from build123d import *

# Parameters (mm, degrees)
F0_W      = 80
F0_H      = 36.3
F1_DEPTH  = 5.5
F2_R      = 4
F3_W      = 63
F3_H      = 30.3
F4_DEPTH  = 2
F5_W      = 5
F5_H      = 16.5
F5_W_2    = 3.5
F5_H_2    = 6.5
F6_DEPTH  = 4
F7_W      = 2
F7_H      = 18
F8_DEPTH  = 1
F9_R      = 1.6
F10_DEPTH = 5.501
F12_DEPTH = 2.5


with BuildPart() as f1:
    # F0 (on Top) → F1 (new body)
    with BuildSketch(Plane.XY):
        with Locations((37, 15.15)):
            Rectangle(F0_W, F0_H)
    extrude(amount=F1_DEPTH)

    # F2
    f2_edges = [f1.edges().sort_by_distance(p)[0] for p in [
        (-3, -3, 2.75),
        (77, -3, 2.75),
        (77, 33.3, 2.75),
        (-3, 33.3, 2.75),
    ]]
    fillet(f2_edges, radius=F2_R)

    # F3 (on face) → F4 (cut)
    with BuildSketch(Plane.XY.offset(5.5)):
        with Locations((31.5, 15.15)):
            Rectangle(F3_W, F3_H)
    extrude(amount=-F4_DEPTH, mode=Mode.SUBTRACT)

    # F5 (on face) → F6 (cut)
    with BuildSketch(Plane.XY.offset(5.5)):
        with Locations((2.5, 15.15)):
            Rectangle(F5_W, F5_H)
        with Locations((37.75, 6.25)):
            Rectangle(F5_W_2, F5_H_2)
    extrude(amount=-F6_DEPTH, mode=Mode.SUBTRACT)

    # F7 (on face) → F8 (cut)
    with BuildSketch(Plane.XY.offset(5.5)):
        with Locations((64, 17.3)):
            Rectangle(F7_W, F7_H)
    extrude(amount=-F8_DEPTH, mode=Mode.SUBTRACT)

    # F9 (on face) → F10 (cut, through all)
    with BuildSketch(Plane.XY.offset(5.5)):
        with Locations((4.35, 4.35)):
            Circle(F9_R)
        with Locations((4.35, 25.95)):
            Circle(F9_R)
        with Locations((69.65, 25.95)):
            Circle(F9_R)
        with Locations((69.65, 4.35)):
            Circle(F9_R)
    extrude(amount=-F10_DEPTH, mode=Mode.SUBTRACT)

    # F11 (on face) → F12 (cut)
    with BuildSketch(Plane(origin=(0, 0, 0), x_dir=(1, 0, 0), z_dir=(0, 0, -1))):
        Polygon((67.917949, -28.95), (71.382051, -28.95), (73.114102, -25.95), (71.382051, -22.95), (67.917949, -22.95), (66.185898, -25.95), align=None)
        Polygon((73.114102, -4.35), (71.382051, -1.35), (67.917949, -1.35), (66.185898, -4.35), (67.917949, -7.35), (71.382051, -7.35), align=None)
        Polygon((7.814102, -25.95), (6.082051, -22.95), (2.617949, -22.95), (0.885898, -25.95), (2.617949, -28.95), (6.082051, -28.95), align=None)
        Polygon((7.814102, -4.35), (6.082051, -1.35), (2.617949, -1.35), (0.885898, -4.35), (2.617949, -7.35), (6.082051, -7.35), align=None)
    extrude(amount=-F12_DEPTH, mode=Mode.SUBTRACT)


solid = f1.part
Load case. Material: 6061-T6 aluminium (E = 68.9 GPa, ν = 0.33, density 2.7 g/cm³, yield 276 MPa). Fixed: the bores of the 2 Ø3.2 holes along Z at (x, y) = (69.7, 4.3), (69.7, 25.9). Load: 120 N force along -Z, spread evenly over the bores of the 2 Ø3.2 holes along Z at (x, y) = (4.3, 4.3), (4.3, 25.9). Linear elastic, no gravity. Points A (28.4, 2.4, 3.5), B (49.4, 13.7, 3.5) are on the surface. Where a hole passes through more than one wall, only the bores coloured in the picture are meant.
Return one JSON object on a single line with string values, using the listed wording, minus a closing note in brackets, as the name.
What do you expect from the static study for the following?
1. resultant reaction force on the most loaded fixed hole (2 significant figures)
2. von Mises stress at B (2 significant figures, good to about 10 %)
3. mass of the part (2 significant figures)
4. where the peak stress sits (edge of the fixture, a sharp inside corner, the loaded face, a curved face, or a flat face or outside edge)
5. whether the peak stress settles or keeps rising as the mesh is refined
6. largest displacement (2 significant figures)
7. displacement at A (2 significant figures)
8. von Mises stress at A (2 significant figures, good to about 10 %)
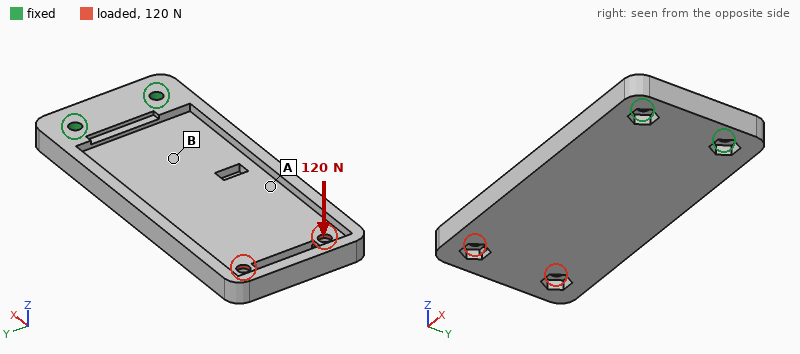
{"resultant reaction force on the most loaded fixed hole": "70 N", "von Mises stress at B": "38 MPa", "mass of the part": "31 g", "where the peak stress sits": "edge of the fixture", "whether the peak stress settles or keeps rising as the mesh is refined": "keeps rising", "largest displacement": "0.94 mm", "displacement at A": "0.39 mm", "von Mises stress at A": "19 MPa"}
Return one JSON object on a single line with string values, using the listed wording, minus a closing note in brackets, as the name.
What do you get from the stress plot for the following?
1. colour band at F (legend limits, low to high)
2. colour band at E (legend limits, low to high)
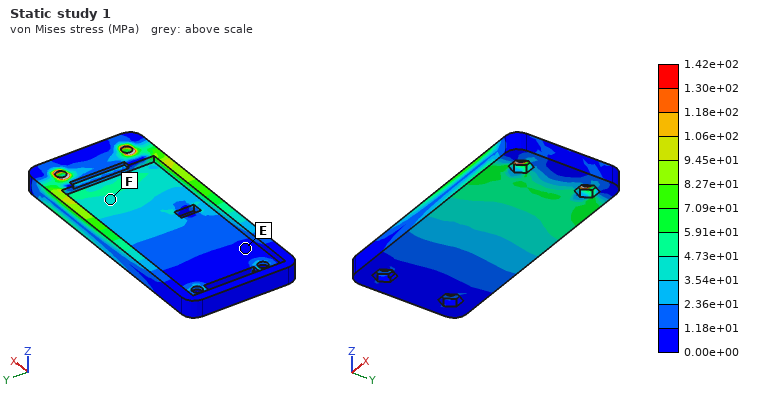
{"colour band at F": "3.54e+01 to 4.73e+01 MPa", "colour band at E": "0.00e+00 to 1.18e+01 MPa"}
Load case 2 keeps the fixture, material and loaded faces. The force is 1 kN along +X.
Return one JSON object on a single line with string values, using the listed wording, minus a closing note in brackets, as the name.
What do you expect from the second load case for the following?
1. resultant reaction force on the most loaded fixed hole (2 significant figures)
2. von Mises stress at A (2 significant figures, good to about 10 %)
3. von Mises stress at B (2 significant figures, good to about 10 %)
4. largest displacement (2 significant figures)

{"resultant reaction force on the most loaded fixed hole": "500 N", "von Mises stress at A": "13 MPa", "von Mises stress at B": "14 MPa", "largest displacement": "0.14 mm"}
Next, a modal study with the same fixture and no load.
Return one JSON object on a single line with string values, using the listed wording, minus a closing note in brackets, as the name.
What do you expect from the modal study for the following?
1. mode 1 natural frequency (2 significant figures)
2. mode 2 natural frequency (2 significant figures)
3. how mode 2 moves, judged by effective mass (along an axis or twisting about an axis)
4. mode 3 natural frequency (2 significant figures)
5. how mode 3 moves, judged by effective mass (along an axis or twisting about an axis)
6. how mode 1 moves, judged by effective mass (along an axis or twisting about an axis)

{"mode 1 natural frequency": "660 Hz", "mode 2 natural frequency": "2200 Hz", "how mode 2 moves, judged by effective mass": "twisting about X", "mode 3 natural frequency": "3900 Hz", "how mode 3 moves, judged by effective mass": "along Z", "how mode 1 moves, judged by effective mass": "along Z"}
